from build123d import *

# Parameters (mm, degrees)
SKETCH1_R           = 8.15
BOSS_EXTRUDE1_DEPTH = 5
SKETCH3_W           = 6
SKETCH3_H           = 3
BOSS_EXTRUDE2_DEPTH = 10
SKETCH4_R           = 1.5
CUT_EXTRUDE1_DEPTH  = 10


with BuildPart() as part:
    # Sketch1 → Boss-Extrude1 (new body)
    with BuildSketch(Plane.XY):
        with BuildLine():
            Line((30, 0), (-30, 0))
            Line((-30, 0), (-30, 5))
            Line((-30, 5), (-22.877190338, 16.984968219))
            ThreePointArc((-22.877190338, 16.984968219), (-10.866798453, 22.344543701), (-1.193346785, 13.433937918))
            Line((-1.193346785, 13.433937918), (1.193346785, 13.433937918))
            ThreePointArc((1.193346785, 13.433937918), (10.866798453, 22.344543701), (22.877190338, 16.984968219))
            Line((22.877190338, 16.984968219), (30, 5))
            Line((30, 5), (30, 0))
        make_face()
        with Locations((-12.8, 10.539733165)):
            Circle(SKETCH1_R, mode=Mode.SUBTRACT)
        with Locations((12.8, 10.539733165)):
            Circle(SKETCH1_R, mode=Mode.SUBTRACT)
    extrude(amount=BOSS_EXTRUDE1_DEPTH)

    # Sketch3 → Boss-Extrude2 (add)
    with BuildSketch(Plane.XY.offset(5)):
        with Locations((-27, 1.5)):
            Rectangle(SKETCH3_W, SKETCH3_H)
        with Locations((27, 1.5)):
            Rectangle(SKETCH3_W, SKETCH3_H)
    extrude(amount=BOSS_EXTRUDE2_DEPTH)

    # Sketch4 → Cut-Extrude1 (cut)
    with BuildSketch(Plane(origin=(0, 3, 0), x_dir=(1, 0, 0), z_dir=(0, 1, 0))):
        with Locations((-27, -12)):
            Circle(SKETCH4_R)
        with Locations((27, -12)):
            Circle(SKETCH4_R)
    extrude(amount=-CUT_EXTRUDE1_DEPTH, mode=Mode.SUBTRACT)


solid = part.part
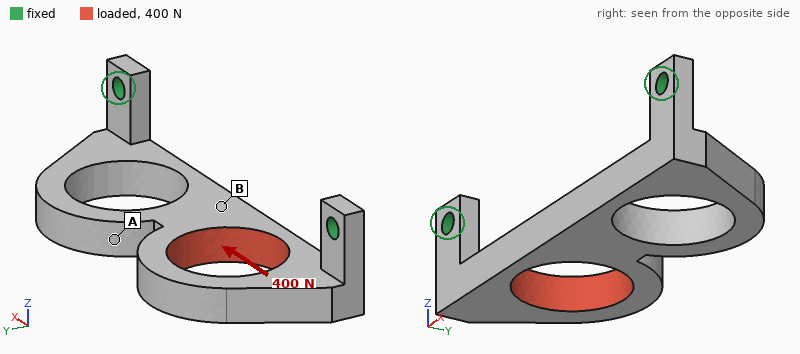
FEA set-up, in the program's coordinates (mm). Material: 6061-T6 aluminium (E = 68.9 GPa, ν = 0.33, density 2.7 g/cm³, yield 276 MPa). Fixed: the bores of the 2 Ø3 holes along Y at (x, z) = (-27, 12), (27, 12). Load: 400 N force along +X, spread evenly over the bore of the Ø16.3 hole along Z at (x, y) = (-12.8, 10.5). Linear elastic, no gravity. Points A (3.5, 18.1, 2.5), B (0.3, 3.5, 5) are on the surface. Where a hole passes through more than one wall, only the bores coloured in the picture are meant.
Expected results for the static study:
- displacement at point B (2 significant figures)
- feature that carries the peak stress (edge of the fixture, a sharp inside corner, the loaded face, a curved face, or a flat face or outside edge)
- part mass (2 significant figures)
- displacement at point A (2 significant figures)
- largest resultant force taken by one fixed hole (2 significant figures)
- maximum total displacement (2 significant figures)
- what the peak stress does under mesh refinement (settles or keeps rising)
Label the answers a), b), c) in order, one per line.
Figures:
a) 20 µm
b) edge of the fixture
c) 9.8 g
d) 22 µm
e) 220 N
f) 36 µm
g) keeps rising
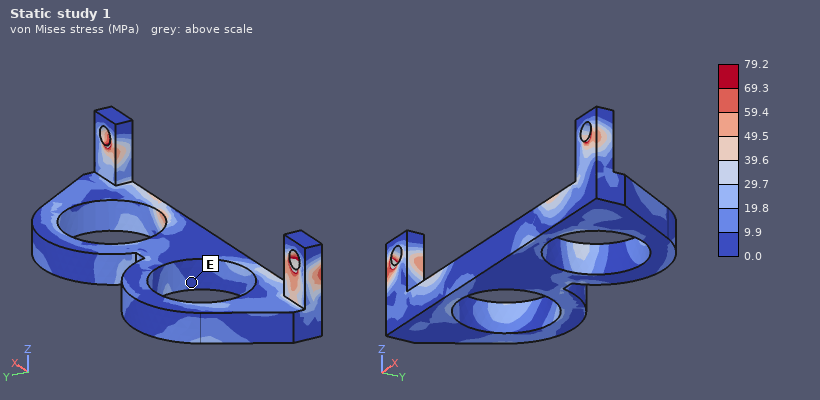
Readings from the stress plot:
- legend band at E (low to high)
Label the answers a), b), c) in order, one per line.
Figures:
a) 0.0 to 9.9 MPa
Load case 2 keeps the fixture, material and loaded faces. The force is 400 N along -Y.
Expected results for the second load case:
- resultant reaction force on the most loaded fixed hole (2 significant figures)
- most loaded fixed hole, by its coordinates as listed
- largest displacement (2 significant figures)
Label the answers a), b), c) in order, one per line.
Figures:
a) 290 N
b) (-27, 12)
c) 0.20 mm
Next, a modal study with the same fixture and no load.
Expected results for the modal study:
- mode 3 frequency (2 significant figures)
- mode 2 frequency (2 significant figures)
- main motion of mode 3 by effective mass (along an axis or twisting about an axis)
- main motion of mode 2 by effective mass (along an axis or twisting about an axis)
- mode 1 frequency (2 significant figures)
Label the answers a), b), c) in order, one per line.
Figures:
a) 5800 Hz
b) 5400 Hz
c) along X
d) along Y
e) 2200 Hz
